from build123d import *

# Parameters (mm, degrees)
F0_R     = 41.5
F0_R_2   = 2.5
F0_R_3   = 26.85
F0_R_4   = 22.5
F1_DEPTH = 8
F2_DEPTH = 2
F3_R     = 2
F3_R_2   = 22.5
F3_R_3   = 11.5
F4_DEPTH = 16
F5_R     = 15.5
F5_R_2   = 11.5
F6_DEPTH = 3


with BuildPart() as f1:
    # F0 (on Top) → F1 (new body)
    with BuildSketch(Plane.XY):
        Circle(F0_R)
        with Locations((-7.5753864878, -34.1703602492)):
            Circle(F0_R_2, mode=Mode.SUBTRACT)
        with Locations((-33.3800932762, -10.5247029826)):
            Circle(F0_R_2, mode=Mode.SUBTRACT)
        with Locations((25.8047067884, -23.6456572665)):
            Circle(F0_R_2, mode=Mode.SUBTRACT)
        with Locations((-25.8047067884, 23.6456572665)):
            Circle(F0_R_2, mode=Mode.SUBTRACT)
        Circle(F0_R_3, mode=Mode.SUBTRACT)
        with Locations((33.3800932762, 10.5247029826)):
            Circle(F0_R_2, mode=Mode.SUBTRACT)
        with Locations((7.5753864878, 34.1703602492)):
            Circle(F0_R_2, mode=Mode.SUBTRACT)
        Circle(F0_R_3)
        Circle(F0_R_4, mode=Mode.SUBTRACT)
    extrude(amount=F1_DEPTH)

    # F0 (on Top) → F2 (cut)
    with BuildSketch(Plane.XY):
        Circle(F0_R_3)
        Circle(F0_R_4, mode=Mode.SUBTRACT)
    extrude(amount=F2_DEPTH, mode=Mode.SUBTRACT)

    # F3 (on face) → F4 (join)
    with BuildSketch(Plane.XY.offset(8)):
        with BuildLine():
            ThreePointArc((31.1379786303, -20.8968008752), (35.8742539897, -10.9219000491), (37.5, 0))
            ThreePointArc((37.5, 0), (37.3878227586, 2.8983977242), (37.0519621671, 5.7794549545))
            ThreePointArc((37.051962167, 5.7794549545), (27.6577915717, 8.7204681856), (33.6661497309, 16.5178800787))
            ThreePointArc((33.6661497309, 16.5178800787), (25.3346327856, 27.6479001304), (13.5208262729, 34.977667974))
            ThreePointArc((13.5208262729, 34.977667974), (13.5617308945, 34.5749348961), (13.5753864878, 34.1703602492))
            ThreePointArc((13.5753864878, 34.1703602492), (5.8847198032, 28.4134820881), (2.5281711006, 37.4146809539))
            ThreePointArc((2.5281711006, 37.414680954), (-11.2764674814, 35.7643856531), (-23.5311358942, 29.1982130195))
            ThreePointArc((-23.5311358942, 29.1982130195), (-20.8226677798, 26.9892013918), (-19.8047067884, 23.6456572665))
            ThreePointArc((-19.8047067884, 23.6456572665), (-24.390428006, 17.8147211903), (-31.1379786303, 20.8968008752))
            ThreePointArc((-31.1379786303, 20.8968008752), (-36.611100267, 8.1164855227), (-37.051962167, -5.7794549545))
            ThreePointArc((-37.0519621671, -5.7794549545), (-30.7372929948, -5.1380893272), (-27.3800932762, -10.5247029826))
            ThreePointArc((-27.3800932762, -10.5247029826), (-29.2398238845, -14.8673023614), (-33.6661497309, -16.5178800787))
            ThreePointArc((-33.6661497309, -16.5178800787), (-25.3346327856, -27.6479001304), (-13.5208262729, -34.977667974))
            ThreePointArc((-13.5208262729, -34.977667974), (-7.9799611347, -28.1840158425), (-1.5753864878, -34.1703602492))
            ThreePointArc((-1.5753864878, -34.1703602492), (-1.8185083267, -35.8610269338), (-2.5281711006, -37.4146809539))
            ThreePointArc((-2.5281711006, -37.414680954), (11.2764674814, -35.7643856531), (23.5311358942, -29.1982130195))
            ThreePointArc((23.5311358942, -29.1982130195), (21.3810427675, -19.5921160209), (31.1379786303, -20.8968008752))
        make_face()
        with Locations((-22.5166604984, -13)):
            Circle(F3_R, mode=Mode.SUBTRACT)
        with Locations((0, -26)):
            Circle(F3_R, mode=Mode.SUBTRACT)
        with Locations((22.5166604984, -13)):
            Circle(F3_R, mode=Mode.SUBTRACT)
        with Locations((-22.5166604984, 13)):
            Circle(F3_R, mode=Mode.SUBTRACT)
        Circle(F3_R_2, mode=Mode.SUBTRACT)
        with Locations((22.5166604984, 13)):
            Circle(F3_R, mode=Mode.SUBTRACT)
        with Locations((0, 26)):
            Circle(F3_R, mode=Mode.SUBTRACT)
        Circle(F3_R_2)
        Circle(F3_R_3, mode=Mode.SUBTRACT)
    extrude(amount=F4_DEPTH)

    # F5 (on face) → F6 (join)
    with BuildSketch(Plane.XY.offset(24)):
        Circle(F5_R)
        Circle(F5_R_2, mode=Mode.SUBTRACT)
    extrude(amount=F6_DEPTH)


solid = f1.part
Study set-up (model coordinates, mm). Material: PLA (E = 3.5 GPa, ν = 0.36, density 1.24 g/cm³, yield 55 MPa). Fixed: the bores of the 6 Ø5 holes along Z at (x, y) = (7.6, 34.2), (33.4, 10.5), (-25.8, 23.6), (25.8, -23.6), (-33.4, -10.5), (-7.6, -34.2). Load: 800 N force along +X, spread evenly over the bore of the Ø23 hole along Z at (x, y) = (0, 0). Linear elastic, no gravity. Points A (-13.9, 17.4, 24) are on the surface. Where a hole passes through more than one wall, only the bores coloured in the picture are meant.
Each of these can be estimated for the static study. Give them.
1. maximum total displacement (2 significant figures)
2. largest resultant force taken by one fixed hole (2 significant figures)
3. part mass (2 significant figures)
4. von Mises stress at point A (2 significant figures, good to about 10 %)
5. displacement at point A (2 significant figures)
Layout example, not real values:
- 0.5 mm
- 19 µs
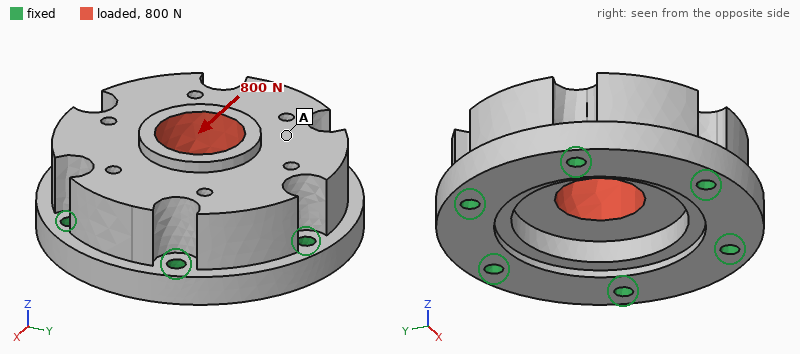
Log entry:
- 17 µm
- 180 N
- 100 g
- 0.43 MPa
- 9.8 µm
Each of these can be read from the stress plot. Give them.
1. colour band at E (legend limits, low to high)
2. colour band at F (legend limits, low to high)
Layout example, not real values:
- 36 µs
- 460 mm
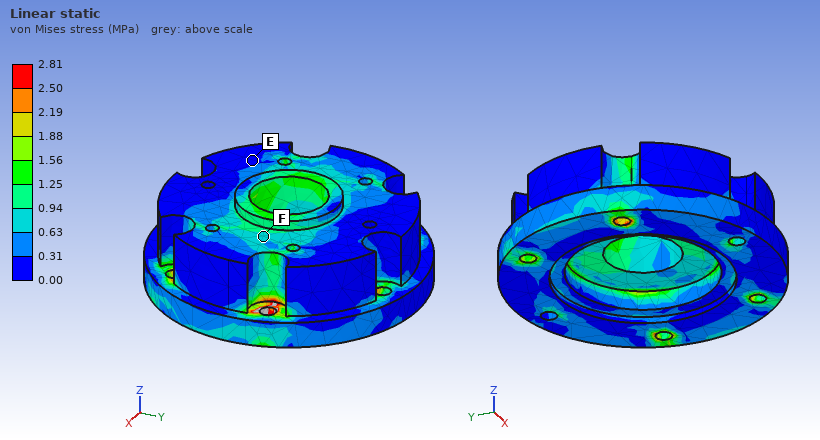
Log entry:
- 0.00 to 0.31 MPa
- 0.63 to 0.94 MPa
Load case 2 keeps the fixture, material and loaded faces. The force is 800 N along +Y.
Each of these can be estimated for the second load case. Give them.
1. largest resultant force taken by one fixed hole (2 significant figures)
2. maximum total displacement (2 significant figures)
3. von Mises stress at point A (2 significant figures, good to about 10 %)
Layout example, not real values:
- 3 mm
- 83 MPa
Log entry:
- 190 N
- 17 µm
- 0.56 MPa
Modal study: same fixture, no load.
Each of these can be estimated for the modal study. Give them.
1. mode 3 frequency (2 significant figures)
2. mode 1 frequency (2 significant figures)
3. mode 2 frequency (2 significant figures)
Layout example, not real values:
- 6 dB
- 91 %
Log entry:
- 5900 Hz
- 5700 Hz
- 5800 Hz
